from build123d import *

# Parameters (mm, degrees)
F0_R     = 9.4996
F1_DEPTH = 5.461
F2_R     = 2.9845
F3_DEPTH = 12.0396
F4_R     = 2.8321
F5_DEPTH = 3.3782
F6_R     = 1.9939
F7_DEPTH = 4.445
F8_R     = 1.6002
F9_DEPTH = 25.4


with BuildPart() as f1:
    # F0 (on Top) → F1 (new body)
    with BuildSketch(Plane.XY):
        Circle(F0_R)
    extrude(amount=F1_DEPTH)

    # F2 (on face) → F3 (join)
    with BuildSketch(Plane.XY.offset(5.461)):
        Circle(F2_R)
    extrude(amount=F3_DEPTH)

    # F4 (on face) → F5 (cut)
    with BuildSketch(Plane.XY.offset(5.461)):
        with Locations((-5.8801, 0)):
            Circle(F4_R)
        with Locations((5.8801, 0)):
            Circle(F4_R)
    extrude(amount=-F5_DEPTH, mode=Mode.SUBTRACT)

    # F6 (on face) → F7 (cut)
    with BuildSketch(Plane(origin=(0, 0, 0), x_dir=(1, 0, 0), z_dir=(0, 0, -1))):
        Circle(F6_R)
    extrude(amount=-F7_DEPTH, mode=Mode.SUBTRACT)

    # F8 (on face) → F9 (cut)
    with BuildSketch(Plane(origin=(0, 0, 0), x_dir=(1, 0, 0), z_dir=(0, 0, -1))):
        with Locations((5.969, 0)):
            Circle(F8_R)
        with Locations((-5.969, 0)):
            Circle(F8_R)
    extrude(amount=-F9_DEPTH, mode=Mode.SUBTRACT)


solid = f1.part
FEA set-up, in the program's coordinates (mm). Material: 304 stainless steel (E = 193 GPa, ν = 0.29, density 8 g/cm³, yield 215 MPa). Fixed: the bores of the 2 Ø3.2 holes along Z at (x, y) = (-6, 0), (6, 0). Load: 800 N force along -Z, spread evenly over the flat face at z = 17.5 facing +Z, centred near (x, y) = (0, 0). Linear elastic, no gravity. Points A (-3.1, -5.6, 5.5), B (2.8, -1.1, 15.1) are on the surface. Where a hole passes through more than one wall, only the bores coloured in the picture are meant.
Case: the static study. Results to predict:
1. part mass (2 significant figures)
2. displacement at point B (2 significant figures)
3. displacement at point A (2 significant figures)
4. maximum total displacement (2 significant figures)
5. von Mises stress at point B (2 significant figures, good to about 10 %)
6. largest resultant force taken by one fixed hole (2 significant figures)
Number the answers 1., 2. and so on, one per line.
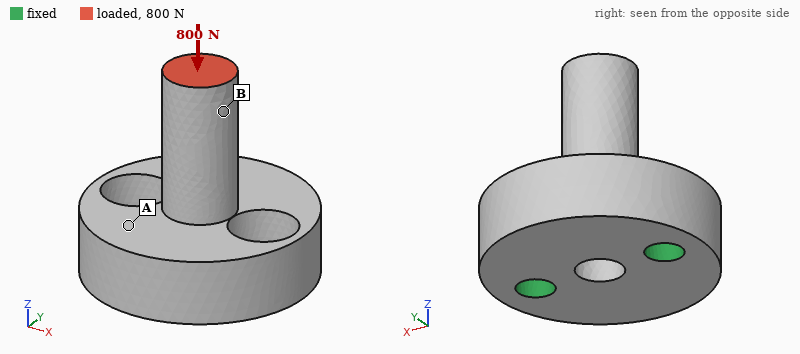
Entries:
1. 13 g
2. 3.0 µm
3. 1.0 µm
4. 3.3 µm
5. 29 MPa
6. 420 N
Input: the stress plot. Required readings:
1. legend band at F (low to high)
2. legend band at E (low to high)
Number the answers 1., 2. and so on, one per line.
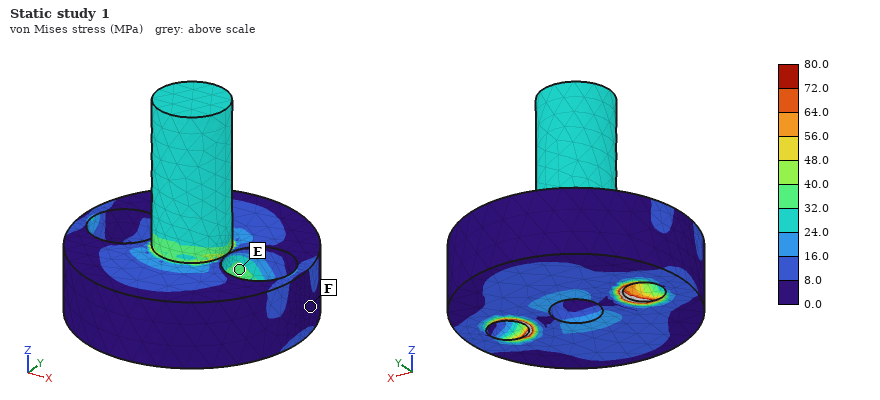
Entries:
1. 0.0 to 8.0 MPa
2. 32.0 to 40.0 MPa
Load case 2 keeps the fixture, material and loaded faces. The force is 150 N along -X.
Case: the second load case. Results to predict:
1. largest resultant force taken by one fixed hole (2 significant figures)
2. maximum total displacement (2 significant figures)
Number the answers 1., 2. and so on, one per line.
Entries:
1. 240 N
2. 15 µm
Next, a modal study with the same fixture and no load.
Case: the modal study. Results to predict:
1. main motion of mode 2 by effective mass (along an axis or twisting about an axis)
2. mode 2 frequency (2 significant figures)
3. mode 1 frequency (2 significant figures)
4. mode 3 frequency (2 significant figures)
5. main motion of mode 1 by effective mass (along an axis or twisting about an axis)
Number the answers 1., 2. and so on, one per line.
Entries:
1. along X
2. 18 kHz
3. 12 kHz
4. 30 kHz
5. along Y
